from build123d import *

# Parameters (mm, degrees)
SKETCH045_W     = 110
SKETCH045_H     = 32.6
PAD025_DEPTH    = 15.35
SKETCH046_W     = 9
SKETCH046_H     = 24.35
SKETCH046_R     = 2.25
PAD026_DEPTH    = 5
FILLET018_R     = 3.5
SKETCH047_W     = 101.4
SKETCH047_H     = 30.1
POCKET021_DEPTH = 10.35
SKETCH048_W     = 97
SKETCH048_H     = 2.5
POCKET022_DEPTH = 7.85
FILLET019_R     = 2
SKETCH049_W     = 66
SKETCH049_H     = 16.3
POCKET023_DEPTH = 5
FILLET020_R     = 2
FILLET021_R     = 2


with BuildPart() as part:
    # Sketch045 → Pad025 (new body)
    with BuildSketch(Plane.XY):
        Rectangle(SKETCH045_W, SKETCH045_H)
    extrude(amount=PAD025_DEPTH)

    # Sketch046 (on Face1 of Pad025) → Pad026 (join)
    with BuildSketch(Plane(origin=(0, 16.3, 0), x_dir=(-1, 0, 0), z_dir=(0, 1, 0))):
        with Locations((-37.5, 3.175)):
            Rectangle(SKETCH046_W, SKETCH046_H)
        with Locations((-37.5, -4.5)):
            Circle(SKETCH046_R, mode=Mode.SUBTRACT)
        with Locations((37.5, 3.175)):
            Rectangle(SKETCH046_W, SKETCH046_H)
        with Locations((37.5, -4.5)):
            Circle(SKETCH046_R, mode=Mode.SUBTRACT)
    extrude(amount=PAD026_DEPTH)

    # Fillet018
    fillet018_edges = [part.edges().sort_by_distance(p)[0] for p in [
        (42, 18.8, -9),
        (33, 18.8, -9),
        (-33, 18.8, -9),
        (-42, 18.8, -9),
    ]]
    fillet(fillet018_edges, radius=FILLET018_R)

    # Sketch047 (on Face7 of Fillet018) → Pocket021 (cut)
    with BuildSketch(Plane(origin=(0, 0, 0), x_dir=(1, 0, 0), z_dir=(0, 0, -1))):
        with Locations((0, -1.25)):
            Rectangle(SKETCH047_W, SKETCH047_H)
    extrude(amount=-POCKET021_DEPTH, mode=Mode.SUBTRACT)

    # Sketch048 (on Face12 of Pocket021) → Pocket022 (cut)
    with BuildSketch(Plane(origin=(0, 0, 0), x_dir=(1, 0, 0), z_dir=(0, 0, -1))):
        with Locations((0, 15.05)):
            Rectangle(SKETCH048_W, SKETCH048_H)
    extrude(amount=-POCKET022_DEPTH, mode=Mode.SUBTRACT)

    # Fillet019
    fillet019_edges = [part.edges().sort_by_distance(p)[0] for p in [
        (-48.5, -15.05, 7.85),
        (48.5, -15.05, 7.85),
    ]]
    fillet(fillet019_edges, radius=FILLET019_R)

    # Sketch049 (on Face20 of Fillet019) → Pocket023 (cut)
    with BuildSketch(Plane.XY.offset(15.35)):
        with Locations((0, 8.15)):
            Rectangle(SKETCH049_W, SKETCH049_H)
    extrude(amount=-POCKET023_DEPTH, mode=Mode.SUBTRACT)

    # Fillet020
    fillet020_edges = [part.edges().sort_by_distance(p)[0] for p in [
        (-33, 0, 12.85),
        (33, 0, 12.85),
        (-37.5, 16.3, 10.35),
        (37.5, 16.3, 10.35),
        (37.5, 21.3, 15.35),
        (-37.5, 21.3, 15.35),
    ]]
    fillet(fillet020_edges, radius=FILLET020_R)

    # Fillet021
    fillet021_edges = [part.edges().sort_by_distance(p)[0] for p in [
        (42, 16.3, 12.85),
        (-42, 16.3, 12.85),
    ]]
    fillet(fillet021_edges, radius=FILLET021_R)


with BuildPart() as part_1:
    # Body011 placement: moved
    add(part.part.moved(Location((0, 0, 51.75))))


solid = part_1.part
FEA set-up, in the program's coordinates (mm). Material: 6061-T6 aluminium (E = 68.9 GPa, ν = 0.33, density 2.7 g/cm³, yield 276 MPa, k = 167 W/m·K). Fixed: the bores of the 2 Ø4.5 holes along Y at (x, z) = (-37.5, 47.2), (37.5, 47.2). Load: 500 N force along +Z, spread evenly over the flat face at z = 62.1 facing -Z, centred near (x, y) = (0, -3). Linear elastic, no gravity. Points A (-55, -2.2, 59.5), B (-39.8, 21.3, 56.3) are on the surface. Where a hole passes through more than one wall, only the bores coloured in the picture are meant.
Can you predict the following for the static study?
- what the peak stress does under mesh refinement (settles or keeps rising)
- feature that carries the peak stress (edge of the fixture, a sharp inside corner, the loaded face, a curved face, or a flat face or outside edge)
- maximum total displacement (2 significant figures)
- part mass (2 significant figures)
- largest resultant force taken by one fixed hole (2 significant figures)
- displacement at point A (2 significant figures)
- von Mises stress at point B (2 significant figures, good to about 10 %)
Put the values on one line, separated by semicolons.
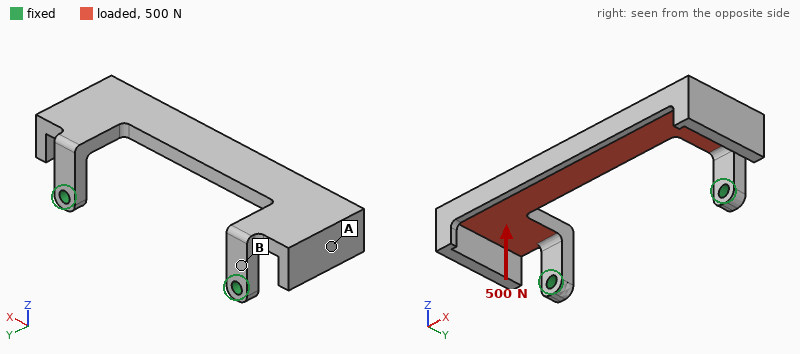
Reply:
keeps rising; edge of the fixture; 0.63 mm; 49 g; 250 N; 0.31 mm; 140 MPa
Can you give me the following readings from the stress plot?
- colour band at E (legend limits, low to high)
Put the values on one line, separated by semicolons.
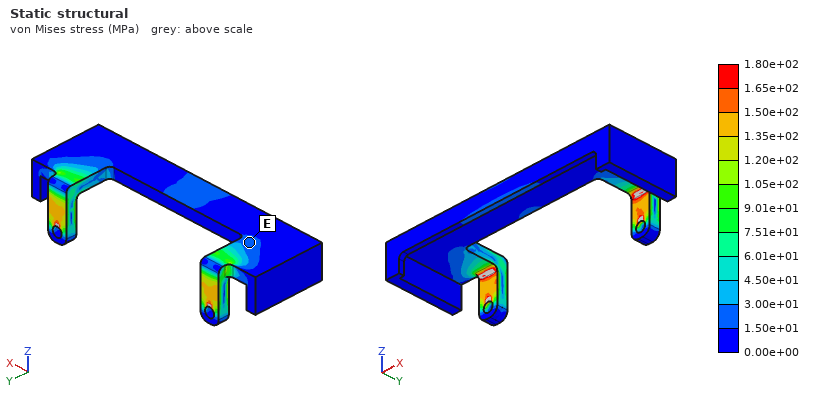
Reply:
1.50e+01 to 3.00e+01 MPa
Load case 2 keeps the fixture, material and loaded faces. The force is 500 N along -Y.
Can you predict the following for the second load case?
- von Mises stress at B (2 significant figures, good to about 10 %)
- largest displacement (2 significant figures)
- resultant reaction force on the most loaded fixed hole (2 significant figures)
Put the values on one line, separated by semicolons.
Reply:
39 MPa; 0.11 mm; 250 N
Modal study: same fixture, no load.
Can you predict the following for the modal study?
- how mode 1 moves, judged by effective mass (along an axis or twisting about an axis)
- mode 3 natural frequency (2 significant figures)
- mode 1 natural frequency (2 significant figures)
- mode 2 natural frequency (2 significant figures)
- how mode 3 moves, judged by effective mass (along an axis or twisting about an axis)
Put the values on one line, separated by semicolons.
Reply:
along Z; 2200 Hz; 790 Hz; 1400 Hz; along X
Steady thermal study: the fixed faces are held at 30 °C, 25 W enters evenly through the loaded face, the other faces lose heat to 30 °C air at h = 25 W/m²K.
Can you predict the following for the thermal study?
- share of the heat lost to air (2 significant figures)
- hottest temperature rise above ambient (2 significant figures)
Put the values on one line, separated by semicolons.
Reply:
23 %; 40 K
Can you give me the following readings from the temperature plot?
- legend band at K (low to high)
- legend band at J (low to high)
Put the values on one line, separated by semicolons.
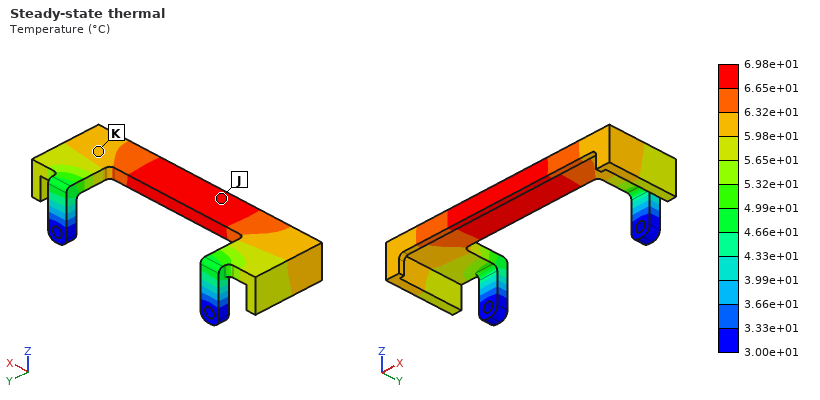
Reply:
5.98e+01 to 6.32e+01 °C; 6.65e+01 to 6.98e+01 °C
